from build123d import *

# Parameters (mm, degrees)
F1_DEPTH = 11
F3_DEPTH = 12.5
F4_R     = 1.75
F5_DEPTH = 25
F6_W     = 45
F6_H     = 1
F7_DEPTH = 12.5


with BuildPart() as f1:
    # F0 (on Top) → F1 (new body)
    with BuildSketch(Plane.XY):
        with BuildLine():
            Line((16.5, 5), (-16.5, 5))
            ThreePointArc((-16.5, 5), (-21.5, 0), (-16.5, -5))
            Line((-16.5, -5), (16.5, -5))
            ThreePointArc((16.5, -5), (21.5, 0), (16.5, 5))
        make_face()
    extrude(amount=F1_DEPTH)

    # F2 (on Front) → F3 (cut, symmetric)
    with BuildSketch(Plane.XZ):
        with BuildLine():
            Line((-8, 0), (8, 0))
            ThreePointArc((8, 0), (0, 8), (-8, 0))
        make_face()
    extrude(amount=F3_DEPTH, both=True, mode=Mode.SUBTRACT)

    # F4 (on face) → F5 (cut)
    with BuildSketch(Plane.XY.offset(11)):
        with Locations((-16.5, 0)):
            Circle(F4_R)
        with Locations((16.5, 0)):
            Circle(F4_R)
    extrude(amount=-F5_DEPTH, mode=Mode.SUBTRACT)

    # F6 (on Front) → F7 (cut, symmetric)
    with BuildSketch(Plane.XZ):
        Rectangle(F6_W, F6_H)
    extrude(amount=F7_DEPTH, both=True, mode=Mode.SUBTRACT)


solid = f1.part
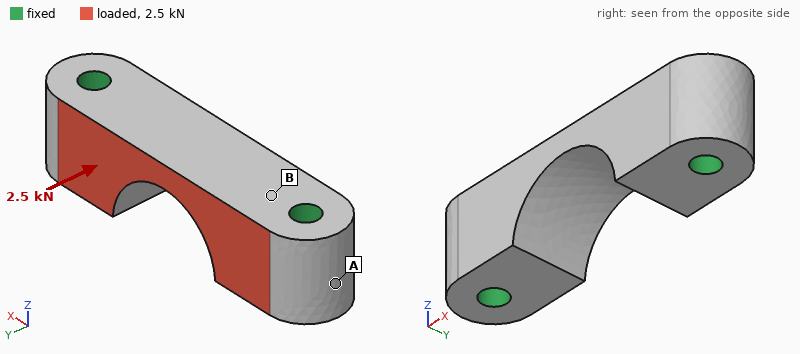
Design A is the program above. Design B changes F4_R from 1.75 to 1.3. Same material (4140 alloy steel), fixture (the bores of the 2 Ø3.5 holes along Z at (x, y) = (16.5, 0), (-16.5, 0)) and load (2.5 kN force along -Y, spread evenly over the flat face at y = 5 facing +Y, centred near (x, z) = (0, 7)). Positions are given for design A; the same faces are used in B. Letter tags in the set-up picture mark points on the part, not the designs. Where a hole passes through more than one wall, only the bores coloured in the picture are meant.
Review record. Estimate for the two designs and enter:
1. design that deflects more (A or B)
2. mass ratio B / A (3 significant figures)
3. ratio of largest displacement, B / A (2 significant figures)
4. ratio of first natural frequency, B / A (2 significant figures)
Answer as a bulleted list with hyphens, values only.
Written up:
- B
- 1.03
- 1.3
- 0.85
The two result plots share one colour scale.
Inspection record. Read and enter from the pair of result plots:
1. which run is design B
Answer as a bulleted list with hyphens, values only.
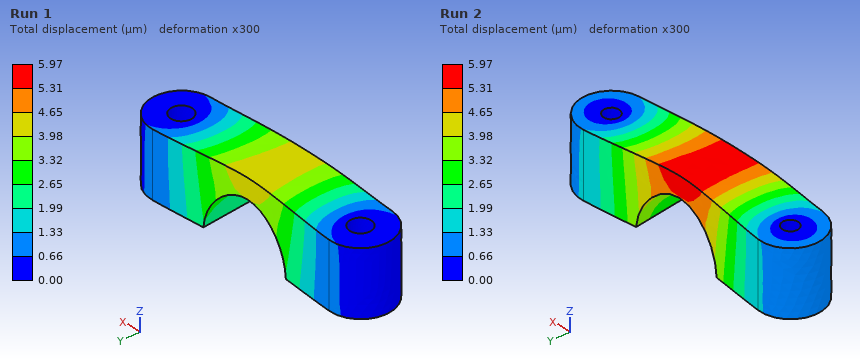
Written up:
- Run 2
